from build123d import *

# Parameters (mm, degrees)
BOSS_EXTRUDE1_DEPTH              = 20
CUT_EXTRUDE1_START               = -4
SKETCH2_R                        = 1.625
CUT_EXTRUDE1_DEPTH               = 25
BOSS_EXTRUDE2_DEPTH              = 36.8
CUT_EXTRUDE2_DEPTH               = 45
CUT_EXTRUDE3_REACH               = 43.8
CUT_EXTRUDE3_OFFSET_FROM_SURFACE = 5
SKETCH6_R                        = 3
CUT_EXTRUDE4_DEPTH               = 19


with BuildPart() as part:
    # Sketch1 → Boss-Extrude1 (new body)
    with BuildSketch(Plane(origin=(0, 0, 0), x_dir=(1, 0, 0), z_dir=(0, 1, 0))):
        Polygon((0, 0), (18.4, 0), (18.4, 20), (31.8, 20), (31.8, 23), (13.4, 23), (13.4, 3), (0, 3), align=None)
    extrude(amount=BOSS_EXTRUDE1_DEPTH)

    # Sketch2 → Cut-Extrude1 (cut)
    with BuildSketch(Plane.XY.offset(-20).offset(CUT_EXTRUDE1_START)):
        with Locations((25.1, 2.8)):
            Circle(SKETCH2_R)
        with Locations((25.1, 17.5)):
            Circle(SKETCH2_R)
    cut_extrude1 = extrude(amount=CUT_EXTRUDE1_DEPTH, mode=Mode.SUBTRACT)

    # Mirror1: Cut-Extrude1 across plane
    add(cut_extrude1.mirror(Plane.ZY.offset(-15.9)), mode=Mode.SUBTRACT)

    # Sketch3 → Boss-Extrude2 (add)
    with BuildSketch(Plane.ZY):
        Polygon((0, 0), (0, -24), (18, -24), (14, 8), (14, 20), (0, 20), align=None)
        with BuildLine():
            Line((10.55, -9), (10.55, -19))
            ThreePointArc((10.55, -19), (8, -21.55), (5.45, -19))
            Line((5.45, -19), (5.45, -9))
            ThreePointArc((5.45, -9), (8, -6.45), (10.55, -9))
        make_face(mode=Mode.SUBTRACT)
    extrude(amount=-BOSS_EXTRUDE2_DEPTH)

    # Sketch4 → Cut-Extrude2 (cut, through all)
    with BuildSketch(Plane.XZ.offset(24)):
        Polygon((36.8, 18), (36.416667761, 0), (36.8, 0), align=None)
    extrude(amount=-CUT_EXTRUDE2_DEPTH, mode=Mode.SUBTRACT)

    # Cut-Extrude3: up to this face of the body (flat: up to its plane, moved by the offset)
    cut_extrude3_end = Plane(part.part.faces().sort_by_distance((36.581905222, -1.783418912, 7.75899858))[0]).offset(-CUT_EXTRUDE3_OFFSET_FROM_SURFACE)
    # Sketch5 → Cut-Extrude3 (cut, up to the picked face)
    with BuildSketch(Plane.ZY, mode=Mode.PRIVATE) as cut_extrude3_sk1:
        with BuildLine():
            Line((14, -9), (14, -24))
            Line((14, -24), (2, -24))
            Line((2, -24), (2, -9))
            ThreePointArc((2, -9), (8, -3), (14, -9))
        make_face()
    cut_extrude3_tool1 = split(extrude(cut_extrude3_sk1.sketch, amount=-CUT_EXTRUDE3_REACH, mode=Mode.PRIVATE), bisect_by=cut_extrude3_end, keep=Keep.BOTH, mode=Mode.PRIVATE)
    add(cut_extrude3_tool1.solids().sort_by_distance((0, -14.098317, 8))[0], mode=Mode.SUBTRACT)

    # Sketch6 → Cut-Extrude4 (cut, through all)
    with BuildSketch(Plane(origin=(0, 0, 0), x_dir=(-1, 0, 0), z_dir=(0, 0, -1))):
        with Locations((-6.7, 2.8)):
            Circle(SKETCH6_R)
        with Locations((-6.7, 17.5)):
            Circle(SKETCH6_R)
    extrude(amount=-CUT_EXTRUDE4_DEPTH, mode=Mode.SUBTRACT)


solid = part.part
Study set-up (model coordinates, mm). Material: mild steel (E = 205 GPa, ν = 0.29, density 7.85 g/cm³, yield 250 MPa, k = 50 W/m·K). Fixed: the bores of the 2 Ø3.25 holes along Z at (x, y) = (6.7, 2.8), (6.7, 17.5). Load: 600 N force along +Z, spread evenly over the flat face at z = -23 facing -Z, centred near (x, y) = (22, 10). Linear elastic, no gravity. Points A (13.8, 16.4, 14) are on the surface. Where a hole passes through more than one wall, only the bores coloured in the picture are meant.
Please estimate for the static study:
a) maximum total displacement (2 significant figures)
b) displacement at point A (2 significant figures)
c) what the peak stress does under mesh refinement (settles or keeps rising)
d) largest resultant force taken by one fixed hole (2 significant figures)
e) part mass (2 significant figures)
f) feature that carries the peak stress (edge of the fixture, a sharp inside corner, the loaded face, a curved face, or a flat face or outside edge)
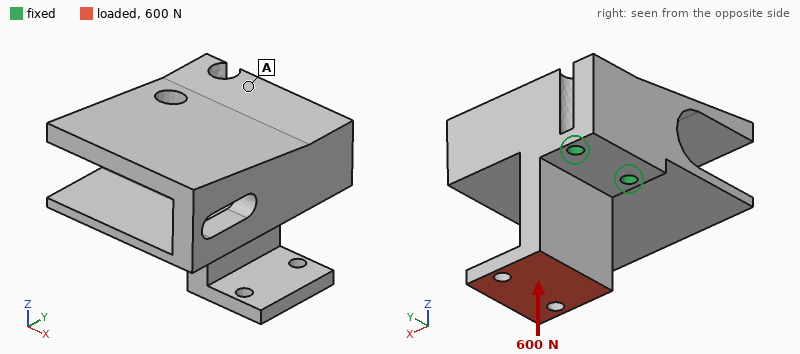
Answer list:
89 µm
16 µm
keeps rising
310 N
160 g
edge of the fixture
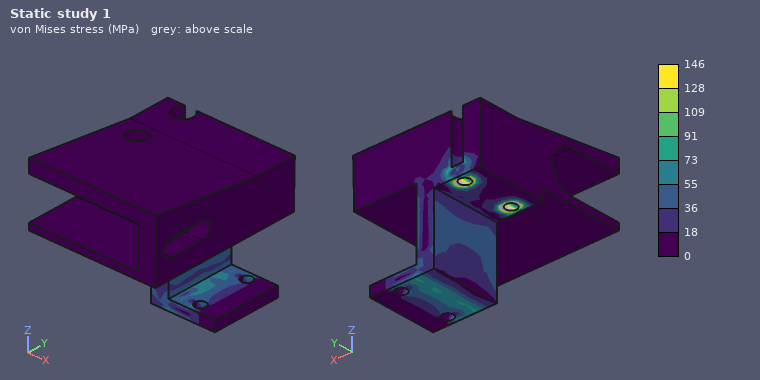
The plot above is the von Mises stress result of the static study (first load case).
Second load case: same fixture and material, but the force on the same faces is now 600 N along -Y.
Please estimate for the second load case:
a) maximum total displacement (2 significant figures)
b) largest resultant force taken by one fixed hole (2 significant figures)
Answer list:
32 µm
1.1 kN
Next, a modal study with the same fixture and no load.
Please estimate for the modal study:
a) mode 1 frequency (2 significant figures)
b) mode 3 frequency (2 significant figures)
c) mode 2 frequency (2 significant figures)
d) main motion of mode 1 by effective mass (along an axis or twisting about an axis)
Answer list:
2000 Hz
5200 Hz
4600 Hz
along Z
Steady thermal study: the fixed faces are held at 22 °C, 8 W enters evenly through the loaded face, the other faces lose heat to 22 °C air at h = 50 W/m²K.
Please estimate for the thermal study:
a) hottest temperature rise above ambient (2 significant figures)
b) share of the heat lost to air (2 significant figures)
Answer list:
46 K
42 %
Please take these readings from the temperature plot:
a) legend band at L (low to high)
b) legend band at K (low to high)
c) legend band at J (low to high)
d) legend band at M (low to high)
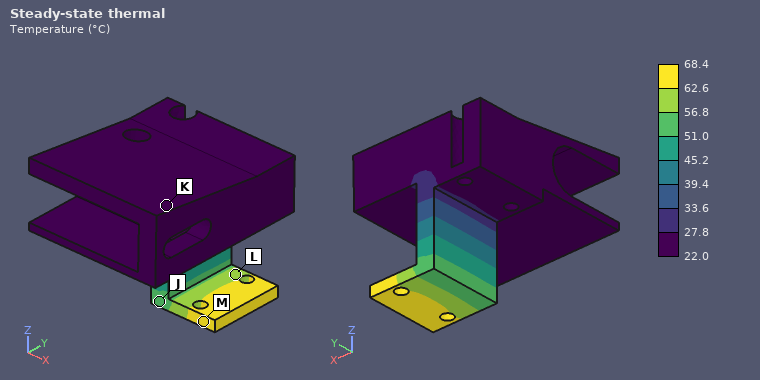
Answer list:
56.8 to 62.6 °C
22.0 to 27.8 °C
51.0 to 56.8 °C
62.6 to 68.4 °C
